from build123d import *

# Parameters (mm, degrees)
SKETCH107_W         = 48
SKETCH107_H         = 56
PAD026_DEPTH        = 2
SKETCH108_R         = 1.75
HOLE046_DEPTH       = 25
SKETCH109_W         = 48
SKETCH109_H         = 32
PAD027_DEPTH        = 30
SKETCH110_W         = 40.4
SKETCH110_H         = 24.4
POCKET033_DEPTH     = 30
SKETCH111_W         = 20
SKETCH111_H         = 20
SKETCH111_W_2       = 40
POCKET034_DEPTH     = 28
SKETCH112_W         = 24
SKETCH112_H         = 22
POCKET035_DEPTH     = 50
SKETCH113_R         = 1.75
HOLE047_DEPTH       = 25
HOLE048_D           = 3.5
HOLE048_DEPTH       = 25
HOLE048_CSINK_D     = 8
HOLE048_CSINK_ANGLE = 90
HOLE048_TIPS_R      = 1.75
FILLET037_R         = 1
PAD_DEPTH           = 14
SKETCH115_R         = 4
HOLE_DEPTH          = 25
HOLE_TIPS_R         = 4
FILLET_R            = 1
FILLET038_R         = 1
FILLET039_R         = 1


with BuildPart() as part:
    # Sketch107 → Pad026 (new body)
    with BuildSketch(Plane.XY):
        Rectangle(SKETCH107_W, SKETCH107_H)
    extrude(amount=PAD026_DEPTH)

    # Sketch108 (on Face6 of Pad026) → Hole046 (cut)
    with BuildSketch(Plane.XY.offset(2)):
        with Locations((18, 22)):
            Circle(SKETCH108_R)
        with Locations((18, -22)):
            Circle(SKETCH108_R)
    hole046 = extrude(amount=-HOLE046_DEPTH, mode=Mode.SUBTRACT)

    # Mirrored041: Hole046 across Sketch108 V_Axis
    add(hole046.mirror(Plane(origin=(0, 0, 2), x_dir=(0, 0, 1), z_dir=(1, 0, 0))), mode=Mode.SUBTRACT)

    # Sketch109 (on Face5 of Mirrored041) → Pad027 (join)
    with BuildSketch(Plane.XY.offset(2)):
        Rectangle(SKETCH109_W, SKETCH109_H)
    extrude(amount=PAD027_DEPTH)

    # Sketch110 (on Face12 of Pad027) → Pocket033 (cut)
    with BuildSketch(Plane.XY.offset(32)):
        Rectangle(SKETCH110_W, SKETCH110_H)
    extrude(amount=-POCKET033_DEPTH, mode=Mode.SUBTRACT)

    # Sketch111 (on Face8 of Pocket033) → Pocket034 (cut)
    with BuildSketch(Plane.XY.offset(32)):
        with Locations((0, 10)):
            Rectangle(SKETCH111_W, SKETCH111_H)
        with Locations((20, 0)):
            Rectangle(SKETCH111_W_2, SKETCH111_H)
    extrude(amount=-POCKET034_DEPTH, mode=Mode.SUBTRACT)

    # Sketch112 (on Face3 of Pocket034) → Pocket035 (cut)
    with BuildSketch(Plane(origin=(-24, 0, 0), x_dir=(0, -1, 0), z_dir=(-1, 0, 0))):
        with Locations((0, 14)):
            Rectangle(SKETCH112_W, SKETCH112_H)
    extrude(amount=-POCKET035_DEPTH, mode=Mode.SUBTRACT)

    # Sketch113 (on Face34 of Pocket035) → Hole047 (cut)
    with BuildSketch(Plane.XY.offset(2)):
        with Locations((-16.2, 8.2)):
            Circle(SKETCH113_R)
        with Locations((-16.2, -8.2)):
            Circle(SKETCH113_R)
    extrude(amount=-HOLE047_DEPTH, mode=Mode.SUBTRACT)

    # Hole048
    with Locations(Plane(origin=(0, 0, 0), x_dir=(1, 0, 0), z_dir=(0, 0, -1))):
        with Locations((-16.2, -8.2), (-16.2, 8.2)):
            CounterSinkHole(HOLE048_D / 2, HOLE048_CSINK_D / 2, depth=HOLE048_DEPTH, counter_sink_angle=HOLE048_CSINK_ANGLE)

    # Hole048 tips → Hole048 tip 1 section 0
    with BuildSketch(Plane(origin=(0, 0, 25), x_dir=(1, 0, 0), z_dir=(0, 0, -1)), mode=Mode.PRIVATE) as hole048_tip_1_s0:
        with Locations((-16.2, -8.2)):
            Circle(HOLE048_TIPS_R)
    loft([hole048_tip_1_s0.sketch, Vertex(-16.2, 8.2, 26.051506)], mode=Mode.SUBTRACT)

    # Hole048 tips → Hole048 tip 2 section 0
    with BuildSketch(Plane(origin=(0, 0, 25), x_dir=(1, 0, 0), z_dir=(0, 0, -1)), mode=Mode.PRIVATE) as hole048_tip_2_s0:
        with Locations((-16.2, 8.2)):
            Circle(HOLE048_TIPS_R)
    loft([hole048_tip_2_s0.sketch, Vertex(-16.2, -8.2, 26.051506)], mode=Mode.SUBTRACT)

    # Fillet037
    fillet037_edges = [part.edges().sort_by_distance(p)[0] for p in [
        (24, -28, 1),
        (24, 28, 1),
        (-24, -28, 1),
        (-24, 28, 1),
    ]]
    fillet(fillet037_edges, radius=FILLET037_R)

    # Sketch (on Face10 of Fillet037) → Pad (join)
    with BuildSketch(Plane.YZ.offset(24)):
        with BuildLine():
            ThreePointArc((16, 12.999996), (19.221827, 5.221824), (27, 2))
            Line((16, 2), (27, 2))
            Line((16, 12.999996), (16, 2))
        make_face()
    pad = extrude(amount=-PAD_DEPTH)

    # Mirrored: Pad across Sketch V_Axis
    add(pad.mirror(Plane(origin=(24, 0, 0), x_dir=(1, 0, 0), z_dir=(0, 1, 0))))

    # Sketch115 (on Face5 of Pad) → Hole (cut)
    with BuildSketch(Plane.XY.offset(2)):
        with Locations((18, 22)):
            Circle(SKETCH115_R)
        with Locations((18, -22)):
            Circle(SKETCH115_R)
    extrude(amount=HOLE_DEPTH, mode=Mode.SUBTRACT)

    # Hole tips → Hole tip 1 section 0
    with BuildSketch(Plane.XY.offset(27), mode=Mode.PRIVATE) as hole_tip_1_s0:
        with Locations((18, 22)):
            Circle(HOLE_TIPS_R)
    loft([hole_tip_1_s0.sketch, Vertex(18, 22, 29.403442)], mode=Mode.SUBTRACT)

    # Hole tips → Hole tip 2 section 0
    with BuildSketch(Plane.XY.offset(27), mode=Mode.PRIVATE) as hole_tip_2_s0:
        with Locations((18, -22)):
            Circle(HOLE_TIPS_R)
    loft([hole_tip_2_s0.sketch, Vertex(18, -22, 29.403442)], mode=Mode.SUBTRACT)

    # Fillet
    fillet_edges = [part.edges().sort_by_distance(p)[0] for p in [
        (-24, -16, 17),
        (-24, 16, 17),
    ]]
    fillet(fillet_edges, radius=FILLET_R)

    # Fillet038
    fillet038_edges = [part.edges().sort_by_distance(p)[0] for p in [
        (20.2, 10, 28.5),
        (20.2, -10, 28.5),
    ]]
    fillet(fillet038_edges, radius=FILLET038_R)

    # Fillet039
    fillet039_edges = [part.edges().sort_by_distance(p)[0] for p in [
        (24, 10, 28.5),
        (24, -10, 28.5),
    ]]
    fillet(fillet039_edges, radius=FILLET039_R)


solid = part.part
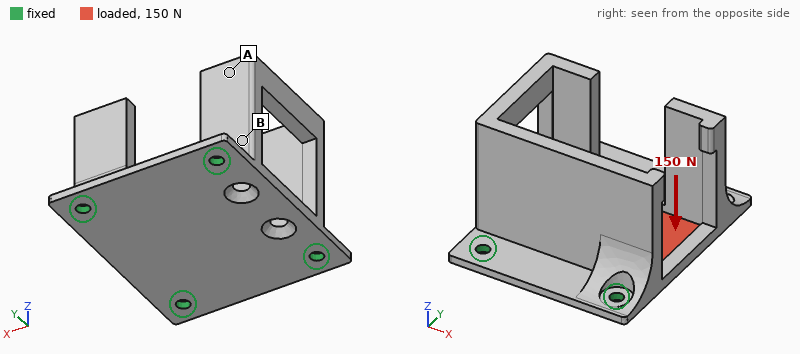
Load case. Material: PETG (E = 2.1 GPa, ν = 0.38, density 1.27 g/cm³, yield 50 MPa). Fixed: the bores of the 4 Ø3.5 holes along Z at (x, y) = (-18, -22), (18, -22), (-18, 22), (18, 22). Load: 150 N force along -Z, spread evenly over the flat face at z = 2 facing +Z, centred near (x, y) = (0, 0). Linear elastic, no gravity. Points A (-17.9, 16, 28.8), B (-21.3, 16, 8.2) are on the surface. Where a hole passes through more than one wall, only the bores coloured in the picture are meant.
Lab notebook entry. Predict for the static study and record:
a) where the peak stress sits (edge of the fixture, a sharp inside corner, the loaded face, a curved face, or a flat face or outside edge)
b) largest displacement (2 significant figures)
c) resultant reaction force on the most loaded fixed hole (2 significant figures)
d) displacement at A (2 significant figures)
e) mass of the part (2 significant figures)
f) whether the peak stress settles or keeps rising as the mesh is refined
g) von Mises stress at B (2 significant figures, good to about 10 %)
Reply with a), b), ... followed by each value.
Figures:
a) edge of the fixture
b) 0.75 mm
c) 45 N
d) 0.24 mm
e) 20 g
f) keeps rising
g) 6.2 MPa
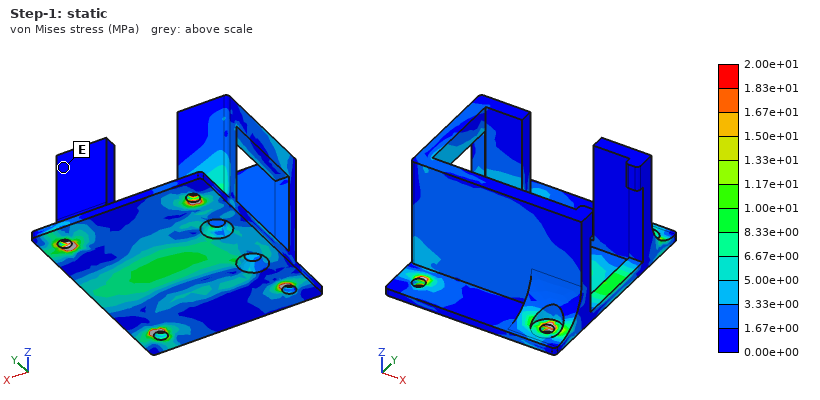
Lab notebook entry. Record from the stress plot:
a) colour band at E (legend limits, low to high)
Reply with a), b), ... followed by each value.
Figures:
a) 0.00e+00 to 1.67e+00 MPa
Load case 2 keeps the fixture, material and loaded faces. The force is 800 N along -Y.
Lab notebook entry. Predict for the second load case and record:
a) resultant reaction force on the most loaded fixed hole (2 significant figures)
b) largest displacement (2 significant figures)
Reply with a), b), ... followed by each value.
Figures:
a) 220 N
b) 0.11 mm
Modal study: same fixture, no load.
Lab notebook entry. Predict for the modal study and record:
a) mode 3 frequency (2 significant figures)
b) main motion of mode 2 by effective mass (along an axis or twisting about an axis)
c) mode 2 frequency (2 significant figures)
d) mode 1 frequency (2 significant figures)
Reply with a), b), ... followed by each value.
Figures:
a) 940 Hz
b) along Y
c) 800 Hz
d) 660 Hz
